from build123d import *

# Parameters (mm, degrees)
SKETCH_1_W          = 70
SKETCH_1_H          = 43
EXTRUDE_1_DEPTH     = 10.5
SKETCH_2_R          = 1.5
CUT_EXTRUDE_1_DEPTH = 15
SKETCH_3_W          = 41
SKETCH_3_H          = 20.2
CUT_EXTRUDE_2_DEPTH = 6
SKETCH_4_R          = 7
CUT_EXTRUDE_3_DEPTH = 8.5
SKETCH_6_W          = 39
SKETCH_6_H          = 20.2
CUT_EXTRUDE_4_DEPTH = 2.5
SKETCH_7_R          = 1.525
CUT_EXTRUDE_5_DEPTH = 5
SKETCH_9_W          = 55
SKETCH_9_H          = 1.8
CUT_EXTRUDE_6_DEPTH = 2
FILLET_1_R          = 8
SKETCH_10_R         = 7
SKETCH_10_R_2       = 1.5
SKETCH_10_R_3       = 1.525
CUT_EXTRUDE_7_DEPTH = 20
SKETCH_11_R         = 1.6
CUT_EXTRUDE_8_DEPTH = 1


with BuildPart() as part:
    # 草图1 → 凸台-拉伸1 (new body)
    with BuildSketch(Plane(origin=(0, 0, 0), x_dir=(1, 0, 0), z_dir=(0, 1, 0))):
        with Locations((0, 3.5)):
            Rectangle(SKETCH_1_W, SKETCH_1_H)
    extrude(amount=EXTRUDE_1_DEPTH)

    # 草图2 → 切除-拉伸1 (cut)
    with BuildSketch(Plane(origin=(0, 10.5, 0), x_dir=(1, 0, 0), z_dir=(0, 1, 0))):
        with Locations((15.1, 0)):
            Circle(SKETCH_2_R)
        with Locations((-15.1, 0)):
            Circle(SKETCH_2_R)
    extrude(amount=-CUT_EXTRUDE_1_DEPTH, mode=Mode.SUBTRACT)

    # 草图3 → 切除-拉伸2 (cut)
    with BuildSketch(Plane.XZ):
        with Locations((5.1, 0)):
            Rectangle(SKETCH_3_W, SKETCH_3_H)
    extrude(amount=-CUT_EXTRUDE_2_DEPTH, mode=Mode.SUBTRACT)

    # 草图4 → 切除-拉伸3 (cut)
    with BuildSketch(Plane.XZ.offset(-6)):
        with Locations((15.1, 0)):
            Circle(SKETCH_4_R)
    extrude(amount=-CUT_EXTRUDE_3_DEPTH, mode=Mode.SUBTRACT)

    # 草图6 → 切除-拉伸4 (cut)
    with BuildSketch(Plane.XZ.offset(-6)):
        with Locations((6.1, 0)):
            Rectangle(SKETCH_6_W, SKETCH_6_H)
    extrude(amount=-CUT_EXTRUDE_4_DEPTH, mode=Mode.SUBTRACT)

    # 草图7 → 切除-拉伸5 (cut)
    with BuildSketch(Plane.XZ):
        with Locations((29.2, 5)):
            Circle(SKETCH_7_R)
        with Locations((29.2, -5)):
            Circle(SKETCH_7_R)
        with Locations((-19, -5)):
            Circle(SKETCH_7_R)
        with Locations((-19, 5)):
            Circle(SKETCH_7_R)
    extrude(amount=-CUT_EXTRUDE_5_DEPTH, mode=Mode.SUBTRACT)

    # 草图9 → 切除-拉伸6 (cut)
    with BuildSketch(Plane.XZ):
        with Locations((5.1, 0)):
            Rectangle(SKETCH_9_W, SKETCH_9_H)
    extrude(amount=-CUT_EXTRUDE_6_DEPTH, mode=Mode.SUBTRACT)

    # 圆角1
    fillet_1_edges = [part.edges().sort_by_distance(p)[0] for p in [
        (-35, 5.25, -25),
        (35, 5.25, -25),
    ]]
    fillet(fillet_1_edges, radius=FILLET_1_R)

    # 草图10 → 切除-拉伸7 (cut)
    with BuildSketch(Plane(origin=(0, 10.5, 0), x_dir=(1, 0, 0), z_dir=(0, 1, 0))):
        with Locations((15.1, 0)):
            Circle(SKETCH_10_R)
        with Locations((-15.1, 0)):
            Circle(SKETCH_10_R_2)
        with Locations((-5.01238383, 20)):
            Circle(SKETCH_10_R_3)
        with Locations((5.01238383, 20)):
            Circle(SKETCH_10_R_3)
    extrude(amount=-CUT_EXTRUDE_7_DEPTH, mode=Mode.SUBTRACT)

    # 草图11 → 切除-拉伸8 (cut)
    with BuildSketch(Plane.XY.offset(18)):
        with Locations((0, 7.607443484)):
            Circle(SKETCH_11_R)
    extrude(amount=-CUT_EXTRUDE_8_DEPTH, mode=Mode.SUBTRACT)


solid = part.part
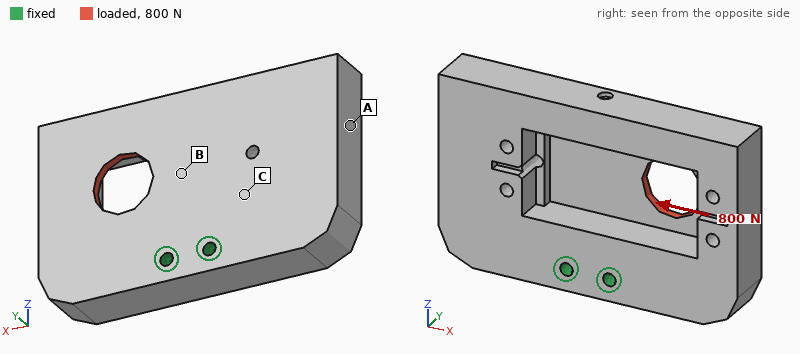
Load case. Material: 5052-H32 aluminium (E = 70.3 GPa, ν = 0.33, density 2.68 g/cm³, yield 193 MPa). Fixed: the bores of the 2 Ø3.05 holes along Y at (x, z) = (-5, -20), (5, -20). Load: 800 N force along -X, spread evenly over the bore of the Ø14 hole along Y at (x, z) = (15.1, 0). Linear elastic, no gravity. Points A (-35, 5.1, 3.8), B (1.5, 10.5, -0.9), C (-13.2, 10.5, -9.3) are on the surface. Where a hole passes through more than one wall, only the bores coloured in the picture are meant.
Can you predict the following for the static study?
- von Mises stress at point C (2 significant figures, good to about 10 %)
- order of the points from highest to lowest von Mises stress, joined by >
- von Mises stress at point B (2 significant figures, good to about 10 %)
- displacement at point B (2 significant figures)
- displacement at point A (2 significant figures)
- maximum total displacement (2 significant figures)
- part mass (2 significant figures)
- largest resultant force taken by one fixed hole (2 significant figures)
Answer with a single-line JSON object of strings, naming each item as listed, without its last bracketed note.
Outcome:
{"von Mises stress at point C": "7.0 MPa", "order of the points from highest to lowest von Mises stress, joined by >": "B > C > A", "von Mises stress at point B": "15 MPa", "displacement at point B": "11 µm", "displacement at point A": "20 µm", "maximum total displacement": "28 µm", "part mass": "63 g", "largest resultant force taken by one fixed hole": "1.3 kN"}
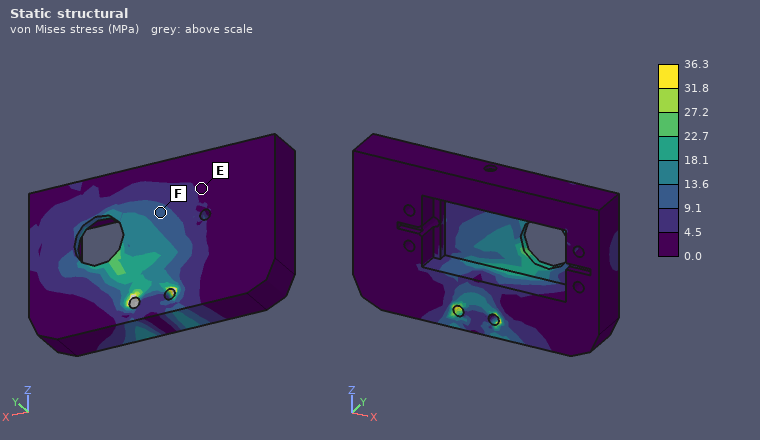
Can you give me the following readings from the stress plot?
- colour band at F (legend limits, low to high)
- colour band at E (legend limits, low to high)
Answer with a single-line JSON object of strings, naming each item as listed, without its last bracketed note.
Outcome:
{"colour band at F": "9.1 to 13.6 MPa", "colour band at E": "0.0 to 4.5 MPa"}
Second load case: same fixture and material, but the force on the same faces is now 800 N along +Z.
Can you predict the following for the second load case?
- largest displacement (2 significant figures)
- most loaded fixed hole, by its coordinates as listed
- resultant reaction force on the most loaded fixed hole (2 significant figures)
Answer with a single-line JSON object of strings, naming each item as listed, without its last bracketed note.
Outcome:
{"largest displacement": "22 µm", "most loaded fixed hole, by its coordinates as listed": "(5, -20)", "resultant reaction force on the most loaded fixed hole": "1.3 kN"}
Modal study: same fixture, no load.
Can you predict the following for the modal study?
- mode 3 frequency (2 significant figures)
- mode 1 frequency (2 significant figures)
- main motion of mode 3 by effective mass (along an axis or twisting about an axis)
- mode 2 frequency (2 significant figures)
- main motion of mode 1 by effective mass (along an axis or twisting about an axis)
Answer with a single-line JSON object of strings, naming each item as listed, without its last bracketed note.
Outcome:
{"mode 3 frequency": "4100 Hz", "mode 1 frequency": "2700 Hz", "main motion of mode 3 by effective mass": "along X", "mode 2 frequency": "3500 Hz", "main motion of mode 1 by effective mass": "along Y"}
